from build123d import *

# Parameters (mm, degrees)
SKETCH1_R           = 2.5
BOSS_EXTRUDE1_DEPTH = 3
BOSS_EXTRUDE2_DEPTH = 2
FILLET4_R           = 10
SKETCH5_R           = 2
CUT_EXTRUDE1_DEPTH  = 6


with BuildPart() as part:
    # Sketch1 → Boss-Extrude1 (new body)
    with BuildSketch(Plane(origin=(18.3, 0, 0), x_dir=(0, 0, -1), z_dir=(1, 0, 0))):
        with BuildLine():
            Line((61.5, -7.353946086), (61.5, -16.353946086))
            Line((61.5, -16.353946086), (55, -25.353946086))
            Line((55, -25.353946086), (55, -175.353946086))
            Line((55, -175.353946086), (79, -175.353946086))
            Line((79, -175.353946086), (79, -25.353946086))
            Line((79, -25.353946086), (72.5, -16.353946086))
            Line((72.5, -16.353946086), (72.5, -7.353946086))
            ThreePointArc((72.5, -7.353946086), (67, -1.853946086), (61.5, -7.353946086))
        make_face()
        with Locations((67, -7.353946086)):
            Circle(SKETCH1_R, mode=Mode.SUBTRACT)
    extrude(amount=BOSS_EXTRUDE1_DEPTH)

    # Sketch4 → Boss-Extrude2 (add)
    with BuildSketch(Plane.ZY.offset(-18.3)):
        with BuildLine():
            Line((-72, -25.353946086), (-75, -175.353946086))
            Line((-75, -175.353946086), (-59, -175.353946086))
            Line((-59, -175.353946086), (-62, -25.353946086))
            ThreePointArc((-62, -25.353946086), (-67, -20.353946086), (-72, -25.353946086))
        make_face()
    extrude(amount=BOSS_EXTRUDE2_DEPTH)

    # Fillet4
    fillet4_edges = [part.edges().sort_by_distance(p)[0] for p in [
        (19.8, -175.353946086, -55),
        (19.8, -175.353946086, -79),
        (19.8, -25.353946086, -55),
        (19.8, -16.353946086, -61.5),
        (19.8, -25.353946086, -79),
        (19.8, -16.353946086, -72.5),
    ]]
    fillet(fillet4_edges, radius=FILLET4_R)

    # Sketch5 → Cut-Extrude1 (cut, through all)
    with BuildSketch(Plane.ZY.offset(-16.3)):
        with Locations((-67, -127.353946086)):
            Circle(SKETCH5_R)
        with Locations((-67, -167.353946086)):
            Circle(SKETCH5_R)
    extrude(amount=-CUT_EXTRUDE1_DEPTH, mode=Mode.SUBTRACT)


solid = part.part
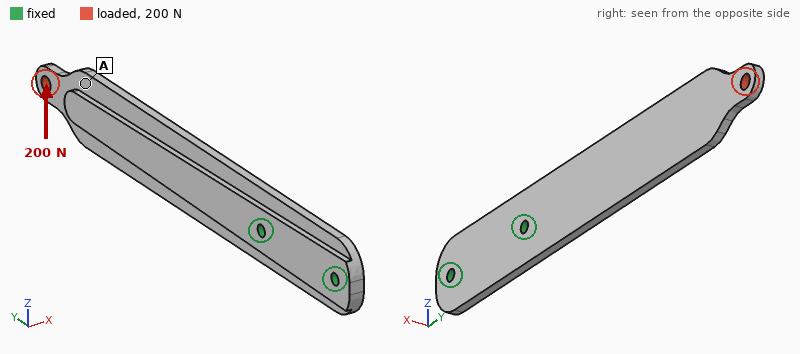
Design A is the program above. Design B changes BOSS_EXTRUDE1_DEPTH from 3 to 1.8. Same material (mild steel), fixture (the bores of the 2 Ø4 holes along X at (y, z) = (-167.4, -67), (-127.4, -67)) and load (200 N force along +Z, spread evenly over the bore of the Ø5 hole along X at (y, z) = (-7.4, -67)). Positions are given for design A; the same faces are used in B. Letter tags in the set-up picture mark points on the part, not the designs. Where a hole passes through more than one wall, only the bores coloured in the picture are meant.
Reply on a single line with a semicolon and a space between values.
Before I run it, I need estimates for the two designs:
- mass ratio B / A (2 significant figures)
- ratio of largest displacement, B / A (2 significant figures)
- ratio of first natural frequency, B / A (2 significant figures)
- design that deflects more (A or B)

0.70; 1.5; 0.81; B
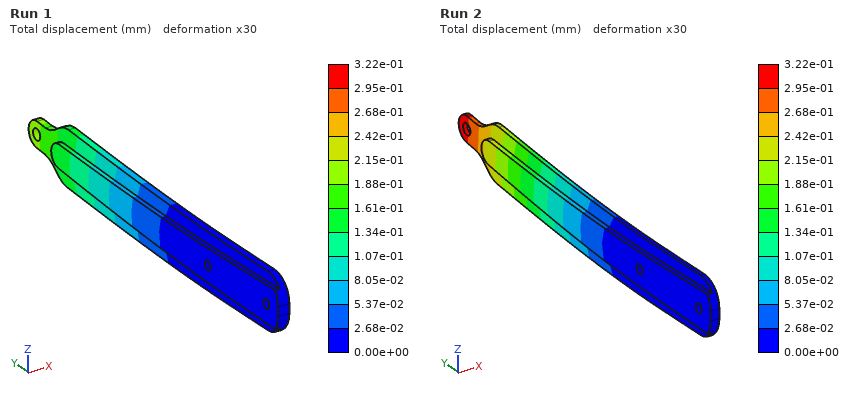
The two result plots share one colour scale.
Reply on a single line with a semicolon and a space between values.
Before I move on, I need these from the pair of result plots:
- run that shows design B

Run 2
